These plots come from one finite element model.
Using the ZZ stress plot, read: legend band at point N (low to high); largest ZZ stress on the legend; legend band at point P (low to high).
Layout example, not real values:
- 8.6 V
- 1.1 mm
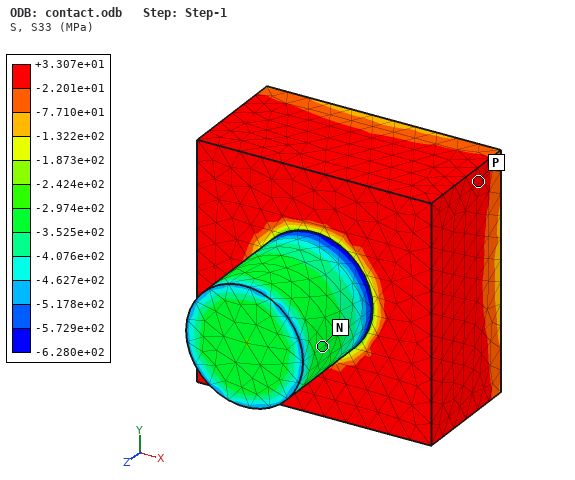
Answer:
- -3.525e+02 to -2.974e+02 MPa
- +3.307e+01 MPa
- -2.201e+01 to +3.307e+01 MPa
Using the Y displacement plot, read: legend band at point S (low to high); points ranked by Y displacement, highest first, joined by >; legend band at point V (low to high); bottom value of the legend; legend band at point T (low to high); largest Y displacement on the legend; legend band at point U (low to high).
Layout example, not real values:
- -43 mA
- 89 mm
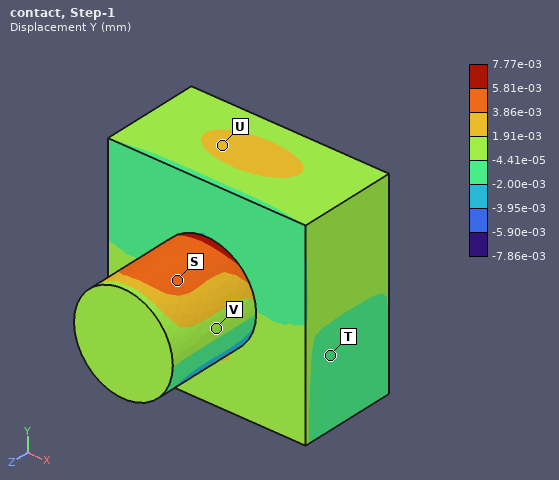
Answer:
- 3.86e-03 to 5.81e-03 mm
- S > U > V > T
- -4.41e-05 to 1.91e-03 mm
- -7.86e-03 mm
- -2.00e-03 to -4.41e-05 mm
- 7.77e-03 mm
- 1.91e-03 to 3.86e-03 mm
